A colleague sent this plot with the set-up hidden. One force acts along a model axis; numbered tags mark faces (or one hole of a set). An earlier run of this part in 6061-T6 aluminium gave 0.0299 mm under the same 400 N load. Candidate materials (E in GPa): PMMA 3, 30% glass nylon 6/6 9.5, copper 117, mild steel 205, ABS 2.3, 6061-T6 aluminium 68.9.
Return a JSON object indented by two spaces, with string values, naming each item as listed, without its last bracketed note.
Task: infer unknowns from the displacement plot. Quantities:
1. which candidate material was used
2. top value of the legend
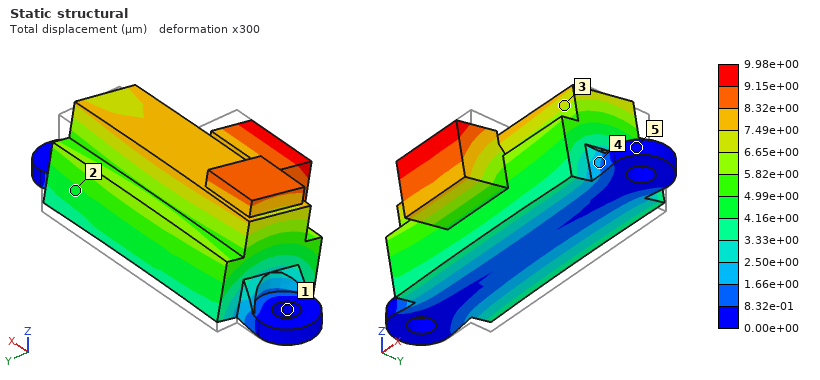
{
  "which candidate material was used": "mild steel",
  "top value of the legend": "9.98e+00 µm"
}
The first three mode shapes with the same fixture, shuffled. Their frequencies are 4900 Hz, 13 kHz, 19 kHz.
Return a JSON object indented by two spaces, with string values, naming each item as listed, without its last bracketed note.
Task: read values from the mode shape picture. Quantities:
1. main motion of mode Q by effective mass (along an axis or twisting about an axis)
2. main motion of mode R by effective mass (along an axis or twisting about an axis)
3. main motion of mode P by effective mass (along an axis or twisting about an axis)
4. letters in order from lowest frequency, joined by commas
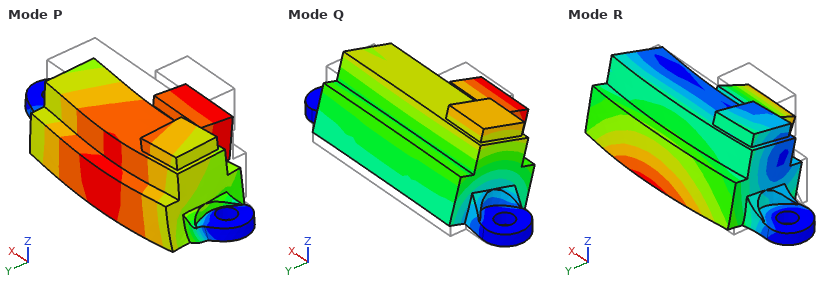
{
  "main motion of mode Q by effective mass": "along Y",
  "main motion of mode R by effective mass": "along Y",
  "main motion of mode P by effective mass": "along Z",
  "letters in order from lowest frequency, joined by commas": "Q, P, R"
}
